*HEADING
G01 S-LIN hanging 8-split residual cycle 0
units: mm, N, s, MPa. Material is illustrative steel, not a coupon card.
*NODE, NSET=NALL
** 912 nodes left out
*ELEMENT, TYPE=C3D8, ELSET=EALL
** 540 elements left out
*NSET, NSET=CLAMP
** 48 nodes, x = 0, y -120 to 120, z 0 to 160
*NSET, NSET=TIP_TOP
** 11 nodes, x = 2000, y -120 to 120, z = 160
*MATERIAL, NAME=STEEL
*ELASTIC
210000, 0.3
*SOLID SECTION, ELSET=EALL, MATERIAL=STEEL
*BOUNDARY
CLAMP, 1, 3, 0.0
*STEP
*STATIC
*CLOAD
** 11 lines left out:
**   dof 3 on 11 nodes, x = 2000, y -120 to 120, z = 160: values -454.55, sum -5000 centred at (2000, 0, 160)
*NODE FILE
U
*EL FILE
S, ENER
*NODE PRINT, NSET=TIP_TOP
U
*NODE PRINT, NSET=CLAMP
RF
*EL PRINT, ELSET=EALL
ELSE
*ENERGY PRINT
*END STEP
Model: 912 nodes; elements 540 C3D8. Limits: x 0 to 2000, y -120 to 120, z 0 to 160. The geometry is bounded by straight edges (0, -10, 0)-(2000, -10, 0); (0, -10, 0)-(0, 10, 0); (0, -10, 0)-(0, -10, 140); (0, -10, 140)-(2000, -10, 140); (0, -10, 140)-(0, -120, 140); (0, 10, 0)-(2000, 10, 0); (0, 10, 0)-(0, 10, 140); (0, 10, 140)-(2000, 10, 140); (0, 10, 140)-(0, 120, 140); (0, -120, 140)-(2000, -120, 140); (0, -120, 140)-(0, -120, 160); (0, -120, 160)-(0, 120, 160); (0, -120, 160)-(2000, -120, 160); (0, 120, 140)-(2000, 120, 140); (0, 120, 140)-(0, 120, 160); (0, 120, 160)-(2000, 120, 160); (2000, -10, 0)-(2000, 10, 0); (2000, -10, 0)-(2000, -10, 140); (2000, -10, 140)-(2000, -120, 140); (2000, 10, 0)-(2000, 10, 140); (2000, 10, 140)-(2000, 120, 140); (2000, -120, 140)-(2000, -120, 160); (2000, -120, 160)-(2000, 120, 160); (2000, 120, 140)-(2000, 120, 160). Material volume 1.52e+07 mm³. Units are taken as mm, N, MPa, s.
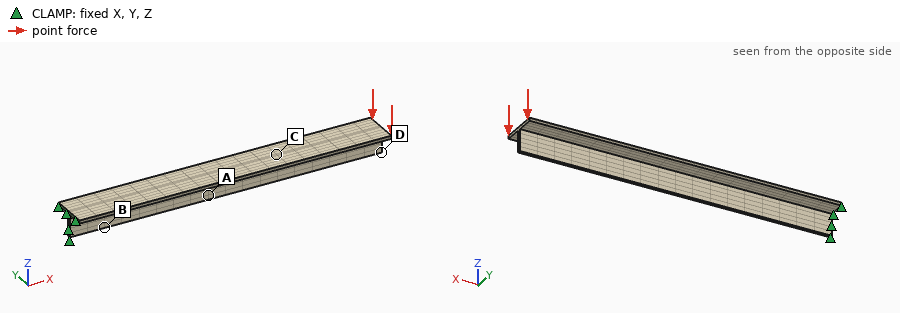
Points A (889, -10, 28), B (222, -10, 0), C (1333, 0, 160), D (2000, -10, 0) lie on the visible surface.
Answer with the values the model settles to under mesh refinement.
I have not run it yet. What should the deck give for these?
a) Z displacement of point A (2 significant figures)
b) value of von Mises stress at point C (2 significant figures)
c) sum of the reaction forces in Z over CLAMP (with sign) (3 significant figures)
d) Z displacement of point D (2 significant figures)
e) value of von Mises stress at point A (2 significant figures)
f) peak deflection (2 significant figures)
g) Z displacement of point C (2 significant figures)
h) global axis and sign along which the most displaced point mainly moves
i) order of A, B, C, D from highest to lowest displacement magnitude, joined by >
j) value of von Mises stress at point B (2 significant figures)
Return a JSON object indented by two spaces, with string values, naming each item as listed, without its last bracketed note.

{
  "Z displacement of point A": "-1.0 mm",
  "value of von Mises stress at point C": "8.2 MPa",
  "sum of the reaction forces in Z over CLAMP (with sign)": "5000 N",
  "Z displacement of point D": "-4.0 mm",
  "value of von Mises stress at point A": "32 MPa",
  "peak deflection": "4.0 mm",
  "Z displacement of point C": "-2.1 mm",
  "global axis and sign along which the most displaced point mainly moves": "-Z",
  "order of A, B, C, D from highest to lowest displacement magnitude, joined by >": "D > C > A > B",
  "value of von Mises stress at point B": "67 MPa"
}
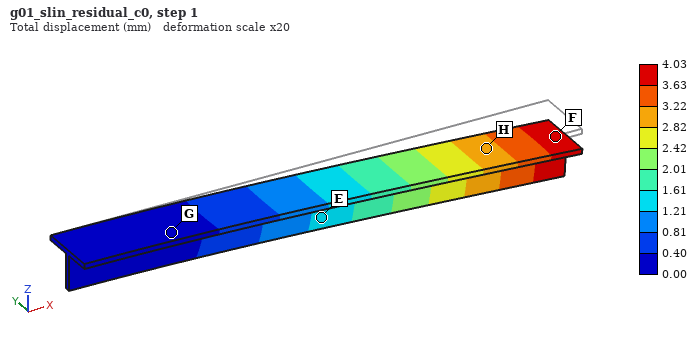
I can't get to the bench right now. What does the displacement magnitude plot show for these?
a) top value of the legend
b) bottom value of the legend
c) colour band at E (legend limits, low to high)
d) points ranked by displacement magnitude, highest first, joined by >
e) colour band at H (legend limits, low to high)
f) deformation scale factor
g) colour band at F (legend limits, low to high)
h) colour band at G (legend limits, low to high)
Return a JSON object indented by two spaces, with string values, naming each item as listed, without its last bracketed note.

{
  "top value of the legend": "4.03 mm",
  "bottom value of the legend": "0.00 mm",
  "colour band at E": "1.21 to 1.61 mm",
  "points ranked by displacement magnitude, highest first, joined by >": "F > H > E > G",
  "colour band at H": "2.82 to 3.22 mm",
  "deformation scale factor": "20",
  "colour band at F": "3.63 to 4.03 mm",
  "colour band at G": "0.00 to 0.40 mm"
}
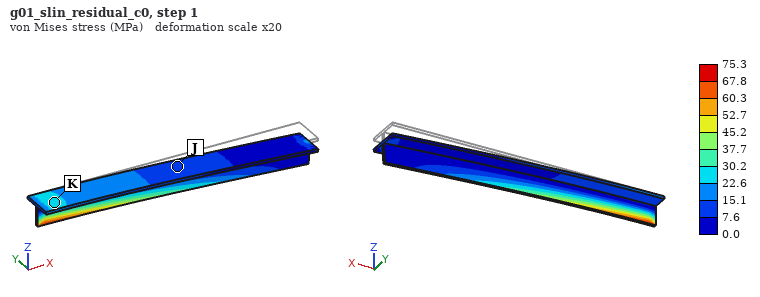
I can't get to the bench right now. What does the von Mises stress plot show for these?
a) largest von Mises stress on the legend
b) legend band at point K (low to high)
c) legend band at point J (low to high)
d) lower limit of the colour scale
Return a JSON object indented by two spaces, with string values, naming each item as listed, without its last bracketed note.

{
  "largest von Mises stress on the legend": "75.3 MPa",
  "legend band at point K": "22.6 to 30.2 MPa",
  "legend band at point J": "7.6 to 15.1 MPa",
  "lower limit of the colour scale": "0.0 MPa"
}
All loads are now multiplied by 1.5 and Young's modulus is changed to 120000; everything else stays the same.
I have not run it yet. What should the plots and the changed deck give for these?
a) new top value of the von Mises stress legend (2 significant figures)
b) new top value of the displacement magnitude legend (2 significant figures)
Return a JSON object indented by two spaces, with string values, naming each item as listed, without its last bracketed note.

{
  "new top value of the von Mises stress legend": "110 MPa",
  "new top value of the displacement magnitude legend": "11 mm"
}
